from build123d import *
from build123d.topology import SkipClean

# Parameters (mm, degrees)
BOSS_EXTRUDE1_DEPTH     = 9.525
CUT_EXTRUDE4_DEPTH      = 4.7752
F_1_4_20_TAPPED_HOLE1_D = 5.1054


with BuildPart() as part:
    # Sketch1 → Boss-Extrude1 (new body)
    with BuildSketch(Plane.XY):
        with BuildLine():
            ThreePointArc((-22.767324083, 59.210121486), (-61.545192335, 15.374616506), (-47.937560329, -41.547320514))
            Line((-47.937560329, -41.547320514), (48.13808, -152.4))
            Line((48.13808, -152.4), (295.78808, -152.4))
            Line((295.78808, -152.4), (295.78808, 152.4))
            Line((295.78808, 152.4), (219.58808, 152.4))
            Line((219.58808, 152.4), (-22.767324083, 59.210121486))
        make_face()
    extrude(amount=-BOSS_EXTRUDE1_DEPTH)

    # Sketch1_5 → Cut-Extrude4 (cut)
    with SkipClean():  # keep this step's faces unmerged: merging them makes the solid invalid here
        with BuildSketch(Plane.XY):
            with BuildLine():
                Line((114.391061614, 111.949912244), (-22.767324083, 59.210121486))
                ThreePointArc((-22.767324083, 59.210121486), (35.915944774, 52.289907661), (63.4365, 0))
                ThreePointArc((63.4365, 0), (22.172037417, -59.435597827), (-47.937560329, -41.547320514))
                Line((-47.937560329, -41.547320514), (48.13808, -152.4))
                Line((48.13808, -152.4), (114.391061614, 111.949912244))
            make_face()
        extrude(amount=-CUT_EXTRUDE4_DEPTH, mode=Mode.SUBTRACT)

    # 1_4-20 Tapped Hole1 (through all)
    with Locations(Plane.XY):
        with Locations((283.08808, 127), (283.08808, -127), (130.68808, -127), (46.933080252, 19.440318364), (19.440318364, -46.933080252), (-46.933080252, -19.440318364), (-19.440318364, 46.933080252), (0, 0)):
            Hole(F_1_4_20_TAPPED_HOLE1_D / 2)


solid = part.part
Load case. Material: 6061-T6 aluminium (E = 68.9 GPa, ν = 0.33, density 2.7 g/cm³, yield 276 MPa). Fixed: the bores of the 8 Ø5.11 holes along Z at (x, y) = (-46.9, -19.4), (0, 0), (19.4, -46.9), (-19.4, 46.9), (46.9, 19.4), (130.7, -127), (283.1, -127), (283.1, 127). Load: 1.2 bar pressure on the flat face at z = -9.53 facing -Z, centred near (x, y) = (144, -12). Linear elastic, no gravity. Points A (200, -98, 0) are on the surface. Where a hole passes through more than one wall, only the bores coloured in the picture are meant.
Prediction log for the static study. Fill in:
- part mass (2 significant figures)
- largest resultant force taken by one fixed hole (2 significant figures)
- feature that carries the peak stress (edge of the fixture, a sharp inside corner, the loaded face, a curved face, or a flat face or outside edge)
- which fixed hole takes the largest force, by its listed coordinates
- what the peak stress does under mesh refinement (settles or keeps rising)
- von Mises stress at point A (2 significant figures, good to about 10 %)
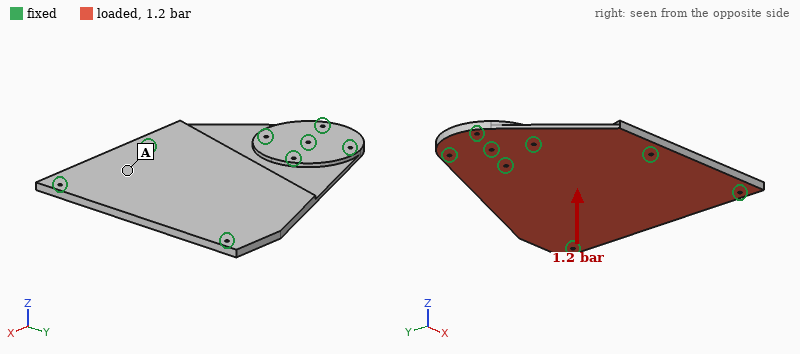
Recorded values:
2.1 kg
3.0 kN
edge of the fixture
(46.9, 19.4)
keeps rising
14 MPa
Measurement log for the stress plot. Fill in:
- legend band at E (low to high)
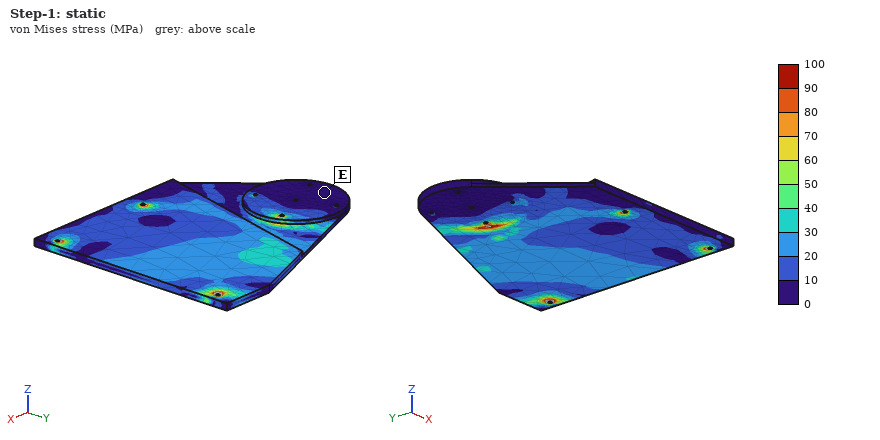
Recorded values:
0 to 10 MPa
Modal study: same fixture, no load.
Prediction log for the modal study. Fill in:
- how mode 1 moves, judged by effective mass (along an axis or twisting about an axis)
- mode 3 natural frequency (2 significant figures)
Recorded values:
along Z
1300 Hz
